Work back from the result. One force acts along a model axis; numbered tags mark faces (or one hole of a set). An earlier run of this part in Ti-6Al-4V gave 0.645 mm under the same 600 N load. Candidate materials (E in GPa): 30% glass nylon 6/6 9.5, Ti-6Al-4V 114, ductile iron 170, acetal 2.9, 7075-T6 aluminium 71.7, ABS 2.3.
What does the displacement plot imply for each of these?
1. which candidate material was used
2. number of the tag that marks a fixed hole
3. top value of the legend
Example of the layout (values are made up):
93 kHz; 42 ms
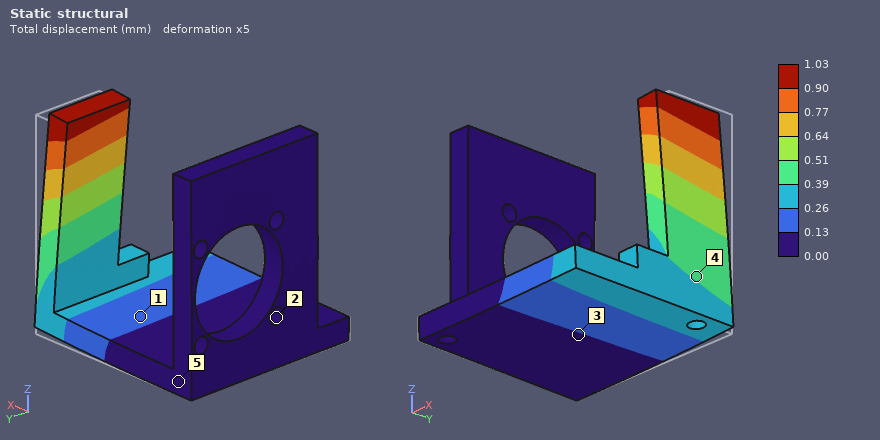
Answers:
7075-T6 aluminium; 2; 1.03 mm
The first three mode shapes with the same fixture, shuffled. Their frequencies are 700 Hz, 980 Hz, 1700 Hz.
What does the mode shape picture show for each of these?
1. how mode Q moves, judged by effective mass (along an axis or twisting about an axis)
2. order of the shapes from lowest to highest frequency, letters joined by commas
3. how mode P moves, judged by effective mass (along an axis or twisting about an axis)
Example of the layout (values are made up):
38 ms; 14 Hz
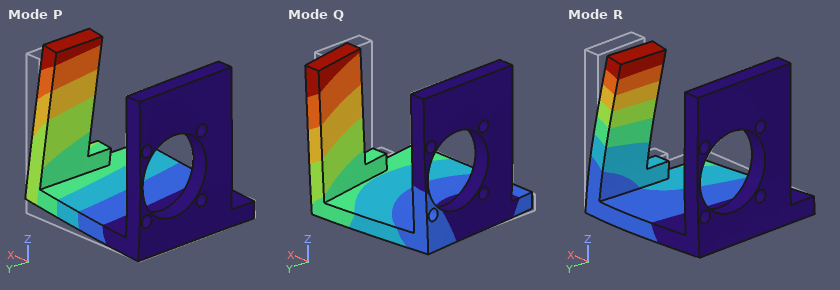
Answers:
along Y; P, Q, R; along Z
